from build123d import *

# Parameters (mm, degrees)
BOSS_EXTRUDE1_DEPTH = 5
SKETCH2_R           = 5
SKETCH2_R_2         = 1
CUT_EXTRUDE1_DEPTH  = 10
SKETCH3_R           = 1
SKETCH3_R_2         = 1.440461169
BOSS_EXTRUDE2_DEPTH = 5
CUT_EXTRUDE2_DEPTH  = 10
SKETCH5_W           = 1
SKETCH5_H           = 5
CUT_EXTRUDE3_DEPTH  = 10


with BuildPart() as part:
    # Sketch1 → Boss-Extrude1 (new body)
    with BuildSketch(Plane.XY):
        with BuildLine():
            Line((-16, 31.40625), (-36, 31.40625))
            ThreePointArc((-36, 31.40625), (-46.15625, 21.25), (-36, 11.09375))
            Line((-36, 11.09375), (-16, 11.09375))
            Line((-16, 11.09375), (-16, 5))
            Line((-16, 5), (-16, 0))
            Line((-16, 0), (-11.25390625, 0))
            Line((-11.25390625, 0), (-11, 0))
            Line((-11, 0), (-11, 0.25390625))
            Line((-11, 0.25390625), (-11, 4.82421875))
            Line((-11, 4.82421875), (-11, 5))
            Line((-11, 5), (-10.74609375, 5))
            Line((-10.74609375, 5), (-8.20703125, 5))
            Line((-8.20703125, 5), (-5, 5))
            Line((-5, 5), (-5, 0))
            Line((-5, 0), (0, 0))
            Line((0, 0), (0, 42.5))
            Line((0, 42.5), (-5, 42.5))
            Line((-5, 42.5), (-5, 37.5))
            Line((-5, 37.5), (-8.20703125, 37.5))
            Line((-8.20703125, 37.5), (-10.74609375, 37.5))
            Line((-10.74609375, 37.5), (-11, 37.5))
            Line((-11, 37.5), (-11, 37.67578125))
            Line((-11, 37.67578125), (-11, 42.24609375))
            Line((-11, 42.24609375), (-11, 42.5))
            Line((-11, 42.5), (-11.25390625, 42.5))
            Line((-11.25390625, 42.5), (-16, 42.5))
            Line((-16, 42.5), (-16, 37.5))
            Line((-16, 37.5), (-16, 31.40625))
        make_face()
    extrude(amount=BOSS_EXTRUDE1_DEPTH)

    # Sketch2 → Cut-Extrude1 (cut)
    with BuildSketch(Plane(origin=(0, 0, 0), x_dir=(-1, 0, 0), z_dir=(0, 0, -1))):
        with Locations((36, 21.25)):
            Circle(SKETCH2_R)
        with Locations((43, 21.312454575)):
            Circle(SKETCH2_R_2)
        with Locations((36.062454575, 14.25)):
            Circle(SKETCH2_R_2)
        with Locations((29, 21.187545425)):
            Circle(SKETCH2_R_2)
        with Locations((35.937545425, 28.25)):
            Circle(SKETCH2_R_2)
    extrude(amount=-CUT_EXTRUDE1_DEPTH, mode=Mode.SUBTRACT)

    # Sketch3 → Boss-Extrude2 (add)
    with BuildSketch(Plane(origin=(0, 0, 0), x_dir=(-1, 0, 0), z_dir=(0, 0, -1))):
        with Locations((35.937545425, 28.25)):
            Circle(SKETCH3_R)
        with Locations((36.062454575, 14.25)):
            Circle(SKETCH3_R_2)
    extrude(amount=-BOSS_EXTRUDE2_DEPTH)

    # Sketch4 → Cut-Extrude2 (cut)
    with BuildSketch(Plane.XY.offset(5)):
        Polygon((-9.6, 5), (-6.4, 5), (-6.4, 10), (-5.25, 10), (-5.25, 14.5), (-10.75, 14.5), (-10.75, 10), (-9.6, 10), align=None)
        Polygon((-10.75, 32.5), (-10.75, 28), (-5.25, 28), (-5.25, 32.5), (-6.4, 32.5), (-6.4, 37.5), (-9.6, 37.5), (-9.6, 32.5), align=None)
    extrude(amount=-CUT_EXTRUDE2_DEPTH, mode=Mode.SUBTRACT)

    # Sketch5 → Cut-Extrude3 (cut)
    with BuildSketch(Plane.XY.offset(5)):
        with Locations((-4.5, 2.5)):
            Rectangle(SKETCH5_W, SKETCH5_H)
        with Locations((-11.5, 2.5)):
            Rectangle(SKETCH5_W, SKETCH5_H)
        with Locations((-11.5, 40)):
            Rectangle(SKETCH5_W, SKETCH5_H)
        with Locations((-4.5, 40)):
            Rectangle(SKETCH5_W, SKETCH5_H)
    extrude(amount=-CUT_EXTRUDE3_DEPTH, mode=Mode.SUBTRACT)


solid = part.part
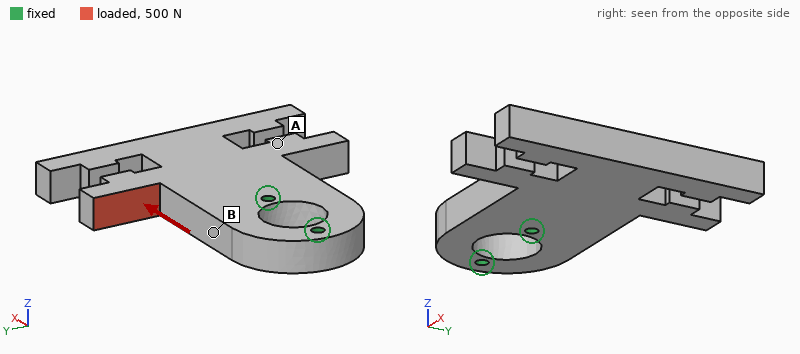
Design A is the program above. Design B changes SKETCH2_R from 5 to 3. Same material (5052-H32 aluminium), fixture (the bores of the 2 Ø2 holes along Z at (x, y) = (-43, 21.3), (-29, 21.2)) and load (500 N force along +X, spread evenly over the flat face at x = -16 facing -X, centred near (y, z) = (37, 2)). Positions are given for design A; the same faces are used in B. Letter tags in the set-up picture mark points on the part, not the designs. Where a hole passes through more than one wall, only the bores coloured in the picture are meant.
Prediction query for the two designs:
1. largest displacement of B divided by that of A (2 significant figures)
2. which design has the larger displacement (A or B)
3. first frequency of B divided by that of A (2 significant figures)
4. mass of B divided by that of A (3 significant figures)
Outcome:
0.92
A
1.0
1.05
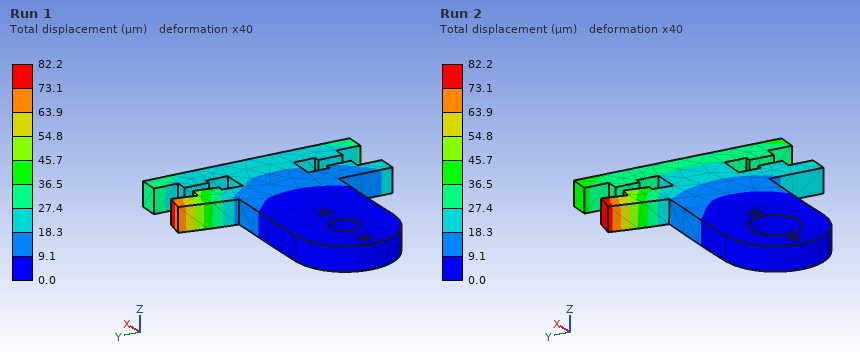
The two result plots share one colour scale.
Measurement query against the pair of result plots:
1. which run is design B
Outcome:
Run 1
